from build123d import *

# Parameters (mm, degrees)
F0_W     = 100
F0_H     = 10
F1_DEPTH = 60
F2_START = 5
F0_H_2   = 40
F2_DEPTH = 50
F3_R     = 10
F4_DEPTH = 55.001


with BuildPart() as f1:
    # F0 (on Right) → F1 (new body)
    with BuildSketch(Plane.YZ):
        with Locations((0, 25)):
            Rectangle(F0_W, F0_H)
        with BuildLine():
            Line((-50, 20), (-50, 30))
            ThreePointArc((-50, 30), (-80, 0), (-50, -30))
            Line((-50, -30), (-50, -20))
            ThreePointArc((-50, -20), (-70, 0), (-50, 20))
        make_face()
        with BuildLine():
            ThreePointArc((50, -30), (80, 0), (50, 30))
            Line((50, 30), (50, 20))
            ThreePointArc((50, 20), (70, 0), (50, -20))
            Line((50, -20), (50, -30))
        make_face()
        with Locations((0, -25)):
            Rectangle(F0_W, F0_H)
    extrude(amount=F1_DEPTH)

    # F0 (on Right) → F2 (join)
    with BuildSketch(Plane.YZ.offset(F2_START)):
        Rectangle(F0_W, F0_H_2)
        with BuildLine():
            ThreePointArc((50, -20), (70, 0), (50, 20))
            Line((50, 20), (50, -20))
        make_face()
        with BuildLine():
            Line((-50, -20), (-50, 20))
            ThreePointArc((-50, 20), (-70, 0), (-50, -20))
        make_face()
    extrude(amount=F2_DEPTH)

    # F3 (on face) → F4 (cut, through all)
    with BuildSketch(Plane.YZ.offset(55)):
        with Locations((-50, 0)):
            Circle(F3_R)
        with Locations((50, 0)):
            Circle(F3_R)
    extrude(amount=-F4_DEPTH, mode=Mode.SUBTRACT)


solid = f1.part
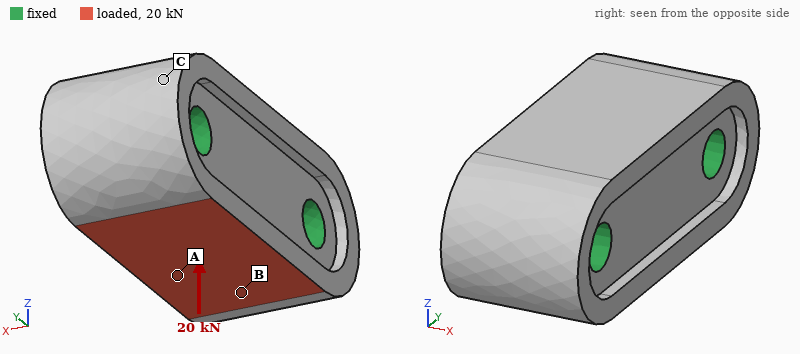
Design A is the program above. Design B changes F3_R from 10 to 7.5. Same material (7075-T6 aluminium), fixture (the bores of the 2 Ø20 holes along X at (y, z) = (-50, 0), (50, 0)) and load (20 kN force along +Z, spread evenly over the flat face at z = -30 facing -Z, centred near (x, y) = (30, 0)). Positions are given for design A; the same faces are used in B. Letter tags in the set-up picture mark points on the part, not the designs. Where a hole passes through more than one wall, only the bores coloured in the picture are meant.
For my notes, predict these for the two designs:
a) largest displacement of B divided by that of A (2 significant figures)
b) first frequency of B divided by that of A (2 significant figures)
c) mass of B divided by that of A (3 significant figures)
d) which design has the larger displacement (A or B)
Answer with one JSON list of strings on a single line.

["1.1", "0.89", "1.03", "B"]
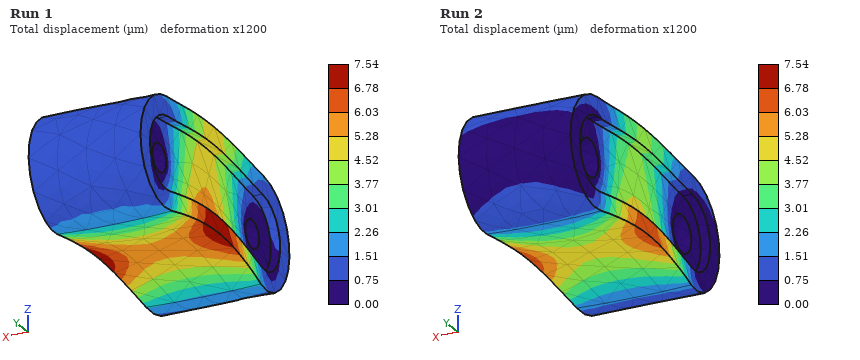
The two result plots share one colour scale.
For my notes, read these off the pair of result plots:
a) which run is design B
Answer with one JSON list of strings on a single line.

["Run 1"]
